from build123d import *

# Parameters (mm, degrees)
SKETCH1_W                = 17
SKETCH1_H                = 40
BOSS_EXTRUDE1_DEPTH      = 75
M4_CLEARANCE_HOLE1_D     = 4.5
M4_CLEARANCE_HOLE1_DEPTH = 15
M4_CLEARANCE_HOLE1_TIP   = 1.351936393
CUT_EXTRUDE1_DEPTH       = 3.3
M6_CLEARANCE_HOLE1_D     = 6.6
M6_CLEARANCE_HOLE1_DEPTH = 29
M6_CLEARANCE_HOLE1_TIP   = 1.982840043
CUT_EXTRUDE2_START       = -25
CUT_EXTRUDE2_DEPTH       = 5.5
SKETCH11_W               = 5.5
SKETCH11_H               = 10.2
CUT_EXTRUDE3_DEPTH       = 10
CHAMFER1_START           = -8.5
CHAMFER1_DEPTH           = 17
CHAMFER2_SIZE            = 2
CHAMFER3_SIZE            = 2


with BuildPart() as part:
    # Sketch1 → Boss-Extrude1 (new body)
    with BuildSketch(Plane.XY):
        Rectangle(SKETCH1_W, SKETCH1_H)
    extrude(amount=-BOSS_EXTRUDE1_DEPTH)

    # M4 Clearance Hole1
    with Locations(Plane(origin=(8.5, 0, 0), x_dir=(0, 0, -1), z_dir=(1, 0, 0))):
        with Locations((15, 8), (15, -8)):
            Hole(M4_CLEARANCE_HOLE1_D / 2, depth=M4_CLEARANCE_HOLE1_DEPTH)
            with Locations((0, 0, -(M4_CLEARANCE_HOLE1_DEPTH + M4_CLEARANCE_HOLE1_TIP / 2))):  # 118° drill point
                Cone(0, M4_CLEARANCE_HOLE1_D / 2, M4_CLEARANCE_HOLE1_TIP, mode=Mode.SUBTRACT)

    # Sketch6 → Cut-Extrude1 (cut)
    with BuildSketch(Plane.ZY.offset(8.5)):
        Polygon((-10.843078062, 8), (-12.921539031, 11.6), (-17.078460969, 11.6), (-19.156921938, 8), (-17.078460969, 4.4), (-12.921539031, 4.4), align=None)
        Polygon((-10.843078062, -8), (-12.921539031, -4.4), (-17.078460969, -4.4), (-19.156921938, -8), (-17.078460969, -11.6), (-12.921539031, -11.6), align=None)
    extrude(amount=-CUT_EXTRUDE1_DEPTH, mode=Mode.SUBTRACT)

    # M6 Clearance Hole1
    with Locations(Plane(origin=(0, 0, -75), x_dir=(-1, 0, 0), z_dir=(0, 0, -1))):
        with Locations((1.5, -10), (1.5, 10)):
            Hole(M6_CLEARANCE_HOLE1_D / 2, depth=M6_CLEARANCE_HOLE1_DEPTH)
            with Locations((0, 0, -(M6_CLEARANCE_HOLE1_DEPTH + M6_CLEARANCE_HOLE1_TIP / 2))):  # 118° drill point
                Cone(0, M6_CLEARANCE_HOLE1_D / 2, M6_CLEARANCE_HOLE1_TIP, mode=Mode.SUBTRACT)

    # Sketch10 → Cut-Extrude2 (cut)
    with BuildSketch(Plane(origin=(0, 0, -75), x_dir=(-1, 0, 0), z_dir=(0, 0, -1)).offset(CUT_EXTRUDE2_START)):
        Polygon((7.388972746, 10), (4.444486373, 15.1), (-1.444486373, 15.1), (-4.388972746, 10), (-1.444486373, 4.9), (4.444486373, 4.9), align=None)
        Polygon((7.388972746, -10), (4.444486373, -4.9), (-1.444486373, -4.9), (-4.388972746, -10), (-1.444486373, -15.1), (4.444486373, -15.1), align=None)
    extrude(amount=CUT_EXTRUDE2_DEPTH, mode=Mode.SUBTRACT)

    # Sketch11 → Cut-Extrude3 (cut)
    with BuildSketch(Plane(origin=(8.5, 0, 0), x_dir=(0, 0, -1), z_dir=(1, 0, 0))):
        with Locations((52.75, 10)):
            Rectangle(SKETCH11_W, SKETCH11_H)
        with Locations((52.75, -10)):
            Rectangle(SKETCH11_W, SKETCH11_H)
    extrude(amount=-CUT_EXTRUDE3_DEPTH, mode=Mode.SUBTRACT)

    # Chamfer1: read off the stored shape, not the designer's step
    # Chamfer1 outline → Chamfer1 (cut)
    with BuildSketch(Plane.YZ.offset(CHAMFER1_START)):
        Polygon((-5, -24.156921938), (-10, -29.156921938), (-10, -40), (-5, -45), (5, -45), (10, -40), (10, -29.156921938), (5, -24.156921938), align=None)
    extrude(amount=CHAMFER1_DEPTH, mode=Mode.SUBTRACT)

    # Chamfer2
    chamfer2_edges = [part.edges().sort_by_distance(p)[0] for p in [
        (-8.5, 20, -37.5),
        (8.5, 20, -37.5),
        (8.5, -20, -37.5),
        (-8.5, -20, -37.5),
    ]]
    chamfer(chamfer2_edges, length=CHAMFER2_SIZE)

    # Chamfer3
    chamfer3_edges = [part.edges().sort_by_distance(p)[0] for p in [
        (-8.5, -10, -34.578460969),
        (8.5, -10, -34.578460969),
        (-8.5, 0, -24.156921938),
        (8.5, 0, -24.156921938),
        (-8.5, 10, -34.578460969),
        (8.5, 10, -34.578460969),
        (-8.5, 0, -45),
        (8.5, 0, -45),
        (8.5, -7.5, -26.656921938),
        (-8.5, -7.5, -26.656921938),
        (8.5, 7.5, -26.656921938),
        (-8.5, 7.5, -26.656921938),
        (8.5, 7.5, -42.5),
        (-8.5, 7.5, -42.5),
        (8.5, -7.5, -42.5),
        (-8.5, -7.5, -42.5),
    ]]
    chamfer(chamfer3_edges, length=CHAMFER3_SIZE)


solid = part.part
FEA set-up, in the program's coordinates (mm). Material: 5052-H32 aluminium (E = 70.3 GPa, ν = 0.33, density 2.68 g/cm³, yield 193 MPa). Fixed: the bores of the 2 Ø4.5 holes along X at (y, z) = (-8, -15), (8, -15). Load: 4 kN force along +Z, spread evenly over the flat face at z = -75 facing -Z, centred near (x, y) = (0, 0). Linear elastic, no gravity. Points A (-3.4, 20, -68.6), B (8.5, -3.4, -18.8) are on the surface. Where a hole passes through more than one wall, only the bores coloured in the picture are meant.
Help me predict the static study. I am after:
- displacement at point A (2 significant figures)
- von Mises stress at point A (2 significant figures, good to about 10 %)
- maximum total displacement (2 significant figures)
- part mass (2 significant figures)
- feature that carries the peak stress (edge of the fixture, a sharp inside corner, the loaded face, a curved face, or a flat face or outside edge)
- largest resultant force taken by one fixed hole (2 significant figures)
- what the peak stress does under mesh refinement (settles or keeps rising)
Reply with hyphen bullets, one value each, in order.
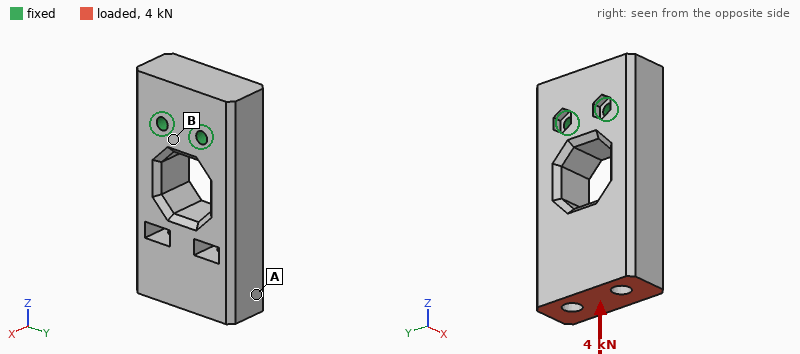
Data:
- 9.6 µm
- 7.6 MPa
- 13 µm
- 110 g
- edge of the fixture
- 2.0 kN
- keeps rising
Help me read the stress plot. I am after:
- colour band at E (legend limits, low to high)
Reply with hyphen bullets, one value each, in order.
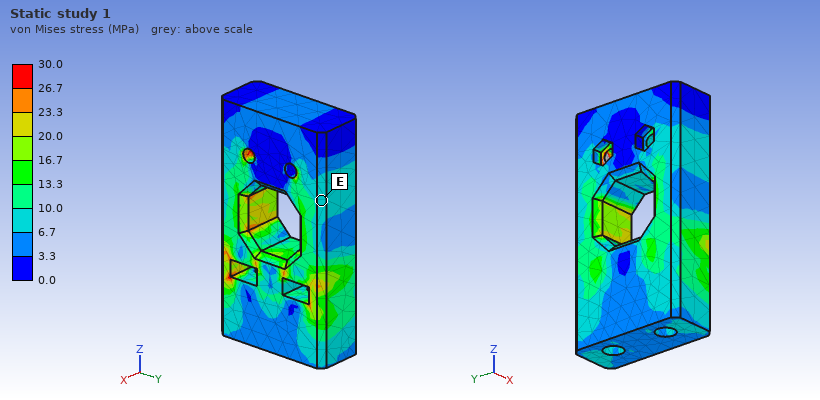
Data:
- 6.7 to 10.0 MPa
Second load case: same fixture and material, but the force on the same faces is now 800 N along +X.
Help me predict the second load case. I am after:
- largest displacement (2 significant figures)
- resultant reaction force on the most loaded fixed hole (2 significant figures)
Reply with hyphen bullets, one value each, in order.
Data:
- 0.12 mm
- 400 N
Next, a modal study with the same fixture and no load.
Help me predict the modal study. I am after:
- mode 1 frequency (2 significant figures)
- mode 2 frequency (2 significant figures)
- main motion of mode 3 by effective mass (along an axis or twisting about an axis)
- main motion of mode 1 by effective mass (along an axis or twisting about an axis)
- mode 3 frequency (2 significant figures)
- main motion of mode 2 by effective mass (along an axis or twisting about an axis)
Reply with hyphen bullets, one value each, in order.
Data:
- 2700 Hz
- 4300 Hz
- twisting about Z
- along X
- 7200 Hz
- along Y
